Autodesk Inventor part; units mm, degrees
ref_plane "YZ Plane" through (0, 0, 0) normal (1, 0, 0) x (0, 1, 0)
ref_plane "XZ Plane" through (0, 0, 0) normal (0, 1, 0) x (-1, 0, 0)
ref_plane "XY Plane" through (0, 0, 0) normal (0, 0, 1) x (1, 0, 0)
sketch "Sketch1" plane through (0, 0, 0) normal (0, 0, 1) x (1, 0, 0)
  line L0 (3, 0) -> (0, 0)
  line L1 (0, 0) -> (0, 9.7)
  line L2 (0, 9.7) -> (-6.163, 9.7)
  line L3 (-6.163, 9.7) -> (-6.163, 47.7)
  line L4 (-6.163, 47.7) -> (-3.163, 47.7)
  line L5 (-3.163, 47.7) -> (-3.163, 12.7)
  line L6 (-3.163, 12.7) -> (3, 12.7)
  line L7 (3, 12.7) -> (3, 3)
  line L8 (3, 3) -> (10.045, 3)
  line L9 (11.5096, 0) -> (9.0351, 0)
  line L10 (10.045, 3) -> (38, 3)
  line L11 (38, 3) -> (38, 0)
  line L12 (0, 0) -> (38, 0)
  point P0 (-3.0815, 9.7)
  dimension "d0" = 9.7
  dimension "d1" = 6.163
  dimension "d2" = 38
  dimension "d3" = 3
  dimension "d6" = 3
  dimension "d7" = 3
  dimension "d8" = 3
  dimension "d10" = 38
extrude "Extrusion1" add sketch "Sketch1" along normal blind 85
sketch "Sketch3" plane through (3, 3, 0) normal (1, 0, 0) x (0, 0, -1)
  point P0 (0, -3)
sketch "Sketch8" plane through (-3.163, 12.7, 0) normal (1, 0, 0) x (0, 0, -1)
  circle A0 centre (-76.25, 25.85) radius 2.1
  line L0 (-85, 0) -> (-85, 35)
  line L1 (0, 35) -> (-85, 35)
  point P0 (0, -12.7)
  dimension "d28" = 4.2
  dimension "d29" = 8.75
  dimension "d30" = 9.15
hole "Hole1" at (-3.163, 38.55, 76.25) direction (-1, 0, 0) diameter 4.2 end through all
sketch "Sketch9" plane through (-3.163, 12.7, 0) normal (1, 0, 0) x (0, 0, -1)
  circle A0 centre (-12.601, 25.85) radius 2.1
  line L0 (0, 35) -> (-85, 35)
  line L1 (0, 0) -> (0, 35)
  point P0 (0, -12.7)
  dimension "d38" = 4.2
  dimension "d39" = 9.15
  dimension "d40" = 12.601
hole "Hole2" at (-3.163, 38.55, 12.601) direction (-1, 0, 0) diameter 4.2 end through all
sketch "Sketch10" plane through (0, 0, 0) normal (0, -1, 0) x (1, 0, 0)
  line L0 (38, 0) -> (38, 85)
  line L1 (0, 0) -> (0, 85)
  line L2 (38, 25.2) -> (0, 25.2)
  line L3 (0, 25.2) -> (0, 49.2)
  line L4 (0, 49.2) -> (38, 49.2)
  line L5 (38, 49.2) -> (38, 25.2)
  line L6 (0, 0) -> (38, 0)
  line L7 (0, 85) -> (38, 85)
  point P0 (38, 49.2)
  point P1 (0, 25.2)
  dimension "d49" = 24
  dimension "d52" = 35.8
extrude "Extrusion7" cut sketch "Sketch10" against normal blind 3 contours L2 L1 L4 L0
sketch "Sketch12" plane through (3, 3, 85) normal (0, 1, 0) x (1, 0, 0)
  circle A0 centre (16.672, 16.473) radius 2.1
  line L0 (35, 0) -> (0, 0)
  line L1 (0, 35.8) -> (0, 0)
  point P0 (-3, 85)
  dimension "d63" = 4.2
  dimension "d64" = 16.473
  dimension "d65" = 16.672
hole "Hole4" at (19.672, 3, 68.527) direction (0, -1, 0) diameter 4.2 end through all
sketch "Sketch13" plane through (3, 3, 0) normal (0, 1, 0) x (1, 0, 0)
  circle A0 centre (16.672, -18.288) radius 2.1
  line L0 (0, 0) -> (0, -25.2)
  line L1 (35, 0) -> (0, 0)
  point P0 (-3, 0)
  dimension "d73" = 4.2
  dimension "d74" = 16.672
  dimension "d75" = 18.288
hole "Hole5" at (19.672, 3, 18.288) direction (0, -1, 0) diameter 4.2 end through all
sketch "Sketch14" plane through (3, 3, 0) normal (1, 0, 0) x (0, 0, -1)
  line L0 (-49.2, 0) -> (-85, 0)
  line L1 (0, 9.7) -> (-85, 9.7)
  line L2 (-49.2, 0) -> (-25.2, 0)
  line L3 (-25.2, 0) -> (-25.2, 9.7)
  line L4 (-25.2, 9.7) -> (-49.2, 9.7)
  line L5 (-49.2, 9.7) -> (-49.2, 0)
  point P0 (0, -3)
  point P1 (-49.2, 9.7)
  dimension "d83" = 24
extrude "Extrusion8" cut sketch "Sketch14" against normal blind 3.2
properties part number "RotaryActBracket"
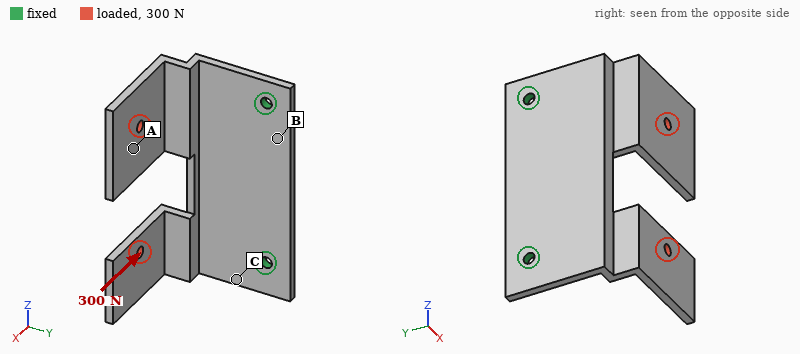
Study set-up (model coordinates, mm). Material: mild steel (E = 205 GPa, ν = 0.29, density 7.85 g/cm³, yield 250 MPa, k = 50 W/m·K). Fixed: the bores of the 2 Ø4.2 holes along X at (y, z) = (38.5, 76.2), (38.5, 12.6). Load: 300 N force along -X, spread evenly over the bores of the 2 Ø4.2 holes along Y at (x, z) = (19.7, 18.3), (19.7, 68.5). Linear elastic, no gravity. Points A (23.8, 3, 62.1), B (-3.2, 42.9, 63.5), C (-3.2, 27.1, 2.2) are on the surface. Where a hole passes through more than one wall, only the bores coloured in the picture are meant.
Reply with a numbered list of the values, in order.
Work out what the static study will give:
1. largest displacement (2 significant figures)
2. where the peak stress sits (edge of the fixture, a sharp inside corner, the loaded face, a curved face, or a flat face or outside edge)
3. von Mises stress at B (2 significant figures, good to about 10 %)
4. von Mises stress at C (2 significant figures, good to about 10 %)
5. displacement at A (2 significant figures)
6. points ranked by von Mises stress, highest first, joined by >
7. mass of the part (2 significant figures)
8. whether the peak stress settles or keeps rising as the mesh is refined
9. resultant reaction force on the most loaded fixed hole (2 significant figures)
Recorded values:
1. 0.38 mm
2. edge of the fixture
3. 49 MPa
4. 81 MPa
5. 0.26 mm
6. C > B > A
7. 150 g
8. keeps rising
9. 160 N
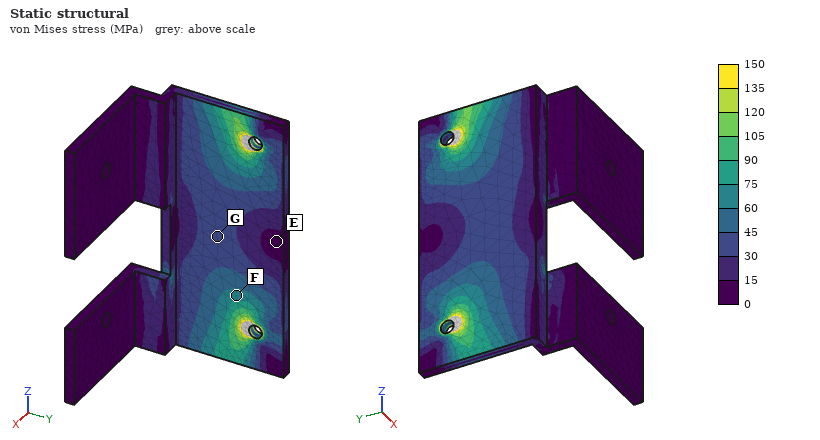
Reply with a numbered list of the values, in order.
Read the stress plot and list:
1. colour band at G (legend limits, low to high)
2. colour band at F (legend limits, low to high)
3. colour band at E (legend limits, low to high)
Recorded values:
1. 30 to 45 MPa
2. 60 to 75 MPa
3. 0 to 15 MPa
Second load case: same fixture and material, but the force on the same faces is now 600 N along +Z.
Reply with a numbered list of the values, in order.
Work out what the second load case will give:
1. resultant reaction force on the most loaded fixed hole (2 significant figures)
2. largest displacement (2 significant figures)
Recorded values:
1. 500 N
2. 0.27 mm
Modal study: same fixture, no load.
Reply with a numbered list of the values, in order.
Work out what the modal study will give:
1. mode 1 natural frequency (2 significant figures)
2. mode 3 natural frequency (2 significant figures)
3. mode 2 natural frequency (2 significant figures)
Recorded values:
1. 550 Hz
2. 1400 Hz
3. 720 Hz
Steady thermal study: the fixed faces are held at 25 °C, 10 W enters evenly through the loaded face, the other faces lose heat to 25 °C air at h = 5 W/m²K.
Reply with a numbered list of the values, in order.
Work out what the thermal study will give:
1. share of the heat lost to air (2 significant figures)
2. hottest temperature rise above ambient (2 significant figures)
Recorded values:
1. 20 %
2. 70 K
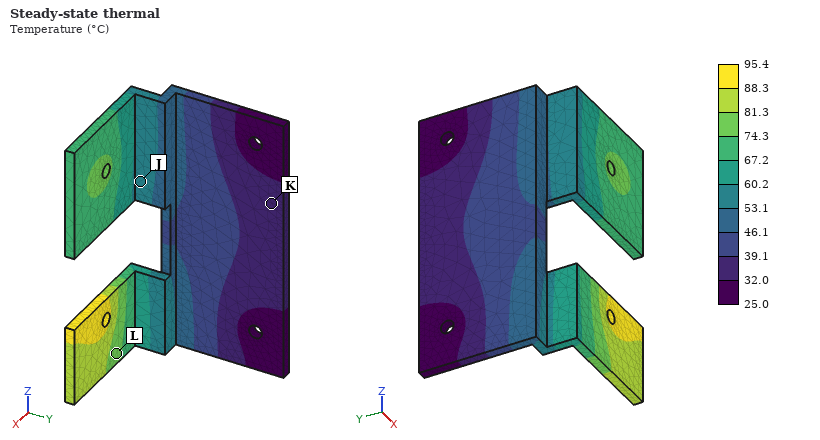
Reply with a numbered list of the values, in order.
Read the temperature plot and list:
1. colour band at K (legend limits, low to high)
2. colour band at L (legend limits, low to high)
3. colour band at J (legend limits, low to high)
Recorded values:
1. 32.0 to 39.1 °C
2. 74.3 to 81.3 °C
3. 53.1 to 60.2 °C
